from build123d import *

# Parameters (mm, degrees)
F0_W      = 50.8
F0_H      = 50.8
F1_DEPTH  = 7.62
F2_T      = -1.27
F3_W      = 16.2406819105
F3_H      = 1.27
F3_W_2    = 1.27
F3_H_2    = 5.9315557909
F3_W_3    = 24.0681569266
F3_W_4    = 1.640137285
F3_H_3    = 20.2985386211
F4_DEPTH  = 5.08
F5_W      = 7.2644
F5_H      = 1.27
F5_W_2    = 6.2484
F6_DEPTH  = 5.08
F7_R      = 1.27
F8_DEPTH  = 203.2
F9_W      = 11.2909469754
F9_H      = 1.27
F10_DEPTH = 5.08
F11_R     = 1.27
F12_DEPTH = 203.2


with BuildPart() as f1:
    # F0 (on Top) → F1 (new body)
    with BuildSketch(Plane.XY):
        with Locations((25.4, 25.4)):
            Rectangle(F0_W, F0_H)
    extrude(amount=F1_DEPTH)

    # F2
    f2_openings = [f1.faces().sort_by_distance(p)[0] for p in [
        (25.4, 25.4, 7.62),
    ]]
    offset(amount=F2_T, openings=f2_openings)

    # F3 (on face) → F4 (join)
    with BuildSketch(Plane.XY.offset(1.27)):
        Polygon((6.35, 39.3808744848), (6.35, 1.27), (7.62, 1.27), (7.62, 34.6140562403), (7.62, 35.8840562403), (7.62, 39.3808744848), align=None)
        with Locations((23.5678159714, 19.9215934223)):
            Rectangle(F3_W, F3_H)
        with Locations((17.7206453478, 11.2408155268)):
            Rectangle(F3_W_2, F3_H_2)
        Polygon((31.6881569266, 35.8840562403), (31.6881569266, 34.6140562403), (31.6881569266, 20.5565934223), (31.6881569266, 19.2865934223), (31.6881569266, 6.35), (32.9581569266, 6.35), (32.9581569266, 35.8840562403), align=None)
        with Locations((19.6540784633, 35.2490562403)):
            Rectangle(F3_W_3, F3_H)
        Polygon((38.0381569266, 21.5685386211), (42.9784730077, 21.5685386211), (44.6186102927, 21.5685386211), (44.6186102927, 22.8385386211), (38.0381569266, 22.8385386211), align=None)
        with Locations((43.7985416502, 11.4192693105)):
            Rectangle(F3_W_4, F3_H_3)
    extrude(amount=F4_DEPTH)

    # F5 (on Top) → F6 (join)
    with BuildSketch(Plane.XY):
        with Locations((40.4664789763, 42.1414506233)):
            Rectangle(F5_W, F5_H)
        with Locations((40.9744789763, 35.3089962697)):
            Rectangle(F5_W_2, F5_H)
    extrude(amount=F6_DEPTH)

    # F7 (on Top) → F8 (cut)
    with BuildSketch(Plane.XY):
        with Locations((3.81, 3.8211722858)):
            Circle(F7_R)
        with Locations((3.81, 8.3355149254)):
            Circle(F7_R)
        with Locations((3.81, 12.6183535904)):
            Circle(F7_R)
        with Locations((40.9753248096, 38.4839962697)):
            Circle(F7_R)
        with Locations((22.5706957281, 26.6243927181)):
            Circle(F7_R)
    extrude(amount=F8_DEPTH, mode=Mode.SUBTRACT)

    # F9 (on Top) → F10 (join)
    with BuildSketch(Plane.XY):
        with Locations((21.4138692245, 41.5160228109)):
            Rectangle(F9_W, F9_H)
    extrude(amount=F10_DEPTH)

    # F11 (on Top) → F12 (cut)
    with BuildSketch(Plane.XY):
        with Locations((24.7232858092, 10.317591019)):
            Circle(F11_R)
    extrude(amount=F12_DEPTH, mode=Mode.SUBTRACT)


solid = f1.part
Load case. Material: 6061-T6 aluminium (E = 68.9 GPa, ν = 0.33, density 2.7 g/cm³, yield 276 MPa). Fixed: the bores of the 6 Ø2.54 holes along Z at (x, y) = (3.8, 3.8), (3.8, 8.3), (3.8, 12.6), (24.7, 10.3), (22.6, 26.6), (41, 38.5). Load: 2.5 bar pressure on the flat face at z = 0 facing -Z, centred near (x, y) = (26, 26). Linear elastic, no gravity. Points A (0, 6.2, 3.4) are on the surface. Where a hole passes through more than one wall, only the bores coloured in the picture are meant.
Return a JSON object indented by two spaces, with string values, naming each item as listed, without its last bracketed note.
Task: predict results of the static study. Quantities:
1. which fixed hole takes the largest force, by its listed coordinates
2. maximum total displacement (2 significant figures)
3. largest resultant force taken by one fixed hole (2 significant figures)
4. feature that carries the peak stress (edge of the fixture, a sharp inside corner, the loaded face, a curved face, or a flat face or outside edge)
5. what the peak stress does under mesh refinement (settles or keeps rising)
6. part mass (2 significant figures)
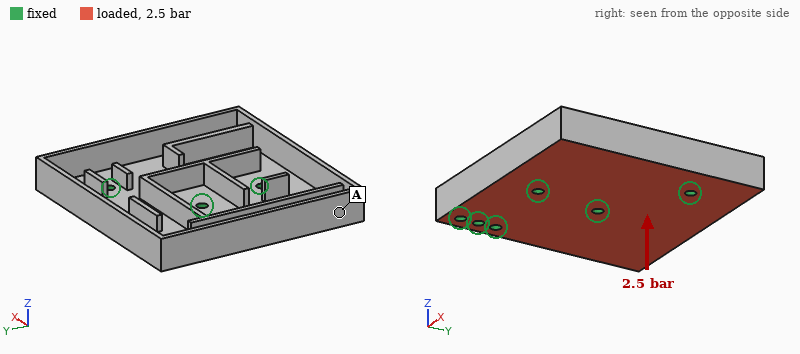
{
  "which fixed hole takes the largest force, by its listed coordinates": "(3.8, 12.6)",
  "maximum total displacement": "0.19 mm",
  "largest resultant force taken by one fixed hole": "300 N",
  "feature that carries the peak stress": "edge of the fixture",
  "what the peak stress does under mesh refinement": "keeps rising",
  "part mass": "16 g"
}
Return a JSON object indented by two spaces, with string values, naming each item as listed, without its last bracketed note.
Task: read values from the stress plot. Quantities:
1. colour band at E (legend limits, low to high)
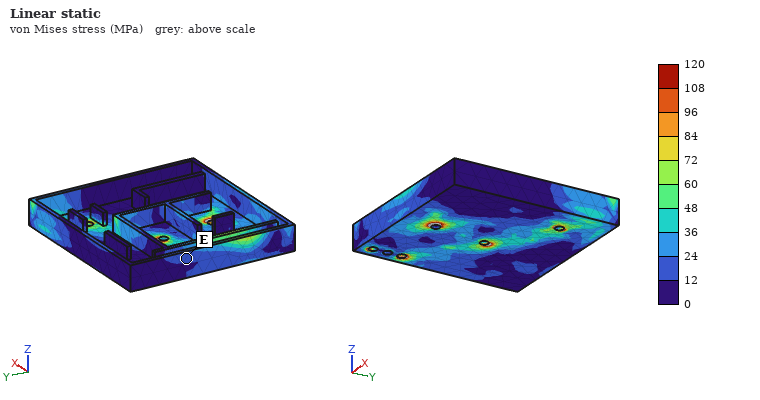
{
  "colour band at E": "12 to 24 MPa"
}
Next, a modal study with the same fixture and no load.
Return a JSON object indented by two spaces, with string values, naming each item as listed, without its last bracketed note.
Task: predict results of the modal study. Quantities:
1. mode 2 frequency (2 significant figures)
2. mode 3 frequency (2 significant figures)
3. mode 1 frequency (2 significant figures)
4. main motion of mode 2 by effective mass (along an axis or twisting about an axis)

{
  "mode 2 frequency": "2900 Hz",
  "mode 3 frequency": "5400 Hz",
  "mode 1 frequency": "2600 Hz",
  "main motion of mode 2 by effective mass": "along Z"
}
